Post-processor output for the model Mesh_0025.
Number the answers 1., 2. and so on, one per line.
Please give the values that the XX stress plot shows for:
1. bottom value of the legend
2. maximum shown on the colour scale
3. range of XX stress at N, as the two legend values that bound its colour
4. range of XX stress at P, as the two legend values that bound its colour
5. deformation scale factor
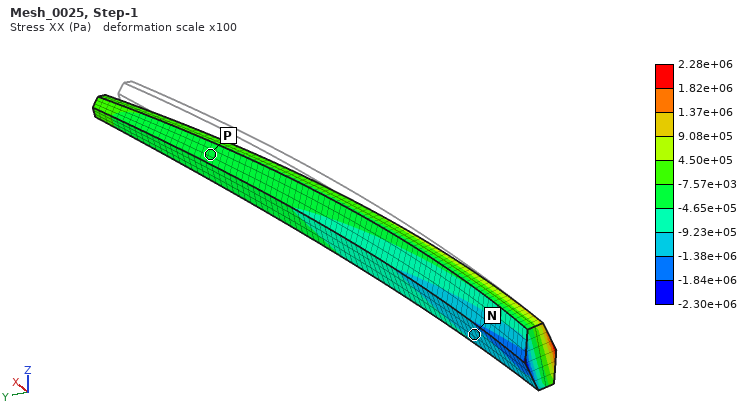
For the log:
1. -2.30e+06 Pa
2. 2.28e+06 Pa
3. -1.38e+06 to -9.23e+05 Pa
4. -4.65e+05 to -7.57e+03 Pa
5. 100
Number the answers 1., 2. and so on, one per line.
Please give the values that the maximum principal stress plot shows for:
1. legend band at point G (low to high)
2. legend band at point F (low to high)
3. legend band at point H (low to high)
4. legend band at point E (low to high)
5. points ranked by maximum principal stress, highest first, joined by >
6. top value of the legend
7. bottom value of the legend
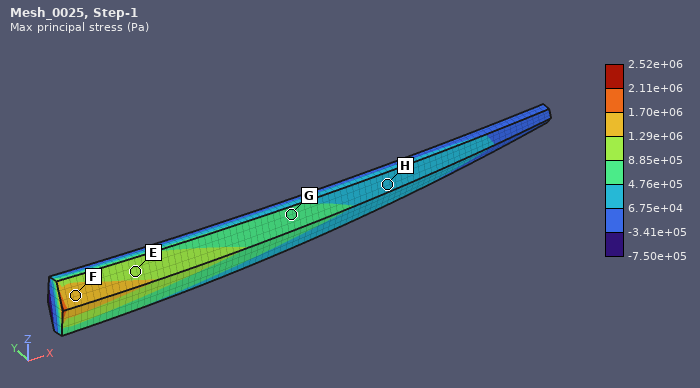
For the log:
1. 4.76e+05 to 8.85e+05 Pa
2. 1.29e+06 to 1.70e+06 Pa
3. 6.75e+04 to 4.76e+05 Pa
4. 8.85e+05 to 1.29e+06 Pa
5. F > E > G > H
6. 2.52e+06 Pa
7. -7.50e+05 Pa
